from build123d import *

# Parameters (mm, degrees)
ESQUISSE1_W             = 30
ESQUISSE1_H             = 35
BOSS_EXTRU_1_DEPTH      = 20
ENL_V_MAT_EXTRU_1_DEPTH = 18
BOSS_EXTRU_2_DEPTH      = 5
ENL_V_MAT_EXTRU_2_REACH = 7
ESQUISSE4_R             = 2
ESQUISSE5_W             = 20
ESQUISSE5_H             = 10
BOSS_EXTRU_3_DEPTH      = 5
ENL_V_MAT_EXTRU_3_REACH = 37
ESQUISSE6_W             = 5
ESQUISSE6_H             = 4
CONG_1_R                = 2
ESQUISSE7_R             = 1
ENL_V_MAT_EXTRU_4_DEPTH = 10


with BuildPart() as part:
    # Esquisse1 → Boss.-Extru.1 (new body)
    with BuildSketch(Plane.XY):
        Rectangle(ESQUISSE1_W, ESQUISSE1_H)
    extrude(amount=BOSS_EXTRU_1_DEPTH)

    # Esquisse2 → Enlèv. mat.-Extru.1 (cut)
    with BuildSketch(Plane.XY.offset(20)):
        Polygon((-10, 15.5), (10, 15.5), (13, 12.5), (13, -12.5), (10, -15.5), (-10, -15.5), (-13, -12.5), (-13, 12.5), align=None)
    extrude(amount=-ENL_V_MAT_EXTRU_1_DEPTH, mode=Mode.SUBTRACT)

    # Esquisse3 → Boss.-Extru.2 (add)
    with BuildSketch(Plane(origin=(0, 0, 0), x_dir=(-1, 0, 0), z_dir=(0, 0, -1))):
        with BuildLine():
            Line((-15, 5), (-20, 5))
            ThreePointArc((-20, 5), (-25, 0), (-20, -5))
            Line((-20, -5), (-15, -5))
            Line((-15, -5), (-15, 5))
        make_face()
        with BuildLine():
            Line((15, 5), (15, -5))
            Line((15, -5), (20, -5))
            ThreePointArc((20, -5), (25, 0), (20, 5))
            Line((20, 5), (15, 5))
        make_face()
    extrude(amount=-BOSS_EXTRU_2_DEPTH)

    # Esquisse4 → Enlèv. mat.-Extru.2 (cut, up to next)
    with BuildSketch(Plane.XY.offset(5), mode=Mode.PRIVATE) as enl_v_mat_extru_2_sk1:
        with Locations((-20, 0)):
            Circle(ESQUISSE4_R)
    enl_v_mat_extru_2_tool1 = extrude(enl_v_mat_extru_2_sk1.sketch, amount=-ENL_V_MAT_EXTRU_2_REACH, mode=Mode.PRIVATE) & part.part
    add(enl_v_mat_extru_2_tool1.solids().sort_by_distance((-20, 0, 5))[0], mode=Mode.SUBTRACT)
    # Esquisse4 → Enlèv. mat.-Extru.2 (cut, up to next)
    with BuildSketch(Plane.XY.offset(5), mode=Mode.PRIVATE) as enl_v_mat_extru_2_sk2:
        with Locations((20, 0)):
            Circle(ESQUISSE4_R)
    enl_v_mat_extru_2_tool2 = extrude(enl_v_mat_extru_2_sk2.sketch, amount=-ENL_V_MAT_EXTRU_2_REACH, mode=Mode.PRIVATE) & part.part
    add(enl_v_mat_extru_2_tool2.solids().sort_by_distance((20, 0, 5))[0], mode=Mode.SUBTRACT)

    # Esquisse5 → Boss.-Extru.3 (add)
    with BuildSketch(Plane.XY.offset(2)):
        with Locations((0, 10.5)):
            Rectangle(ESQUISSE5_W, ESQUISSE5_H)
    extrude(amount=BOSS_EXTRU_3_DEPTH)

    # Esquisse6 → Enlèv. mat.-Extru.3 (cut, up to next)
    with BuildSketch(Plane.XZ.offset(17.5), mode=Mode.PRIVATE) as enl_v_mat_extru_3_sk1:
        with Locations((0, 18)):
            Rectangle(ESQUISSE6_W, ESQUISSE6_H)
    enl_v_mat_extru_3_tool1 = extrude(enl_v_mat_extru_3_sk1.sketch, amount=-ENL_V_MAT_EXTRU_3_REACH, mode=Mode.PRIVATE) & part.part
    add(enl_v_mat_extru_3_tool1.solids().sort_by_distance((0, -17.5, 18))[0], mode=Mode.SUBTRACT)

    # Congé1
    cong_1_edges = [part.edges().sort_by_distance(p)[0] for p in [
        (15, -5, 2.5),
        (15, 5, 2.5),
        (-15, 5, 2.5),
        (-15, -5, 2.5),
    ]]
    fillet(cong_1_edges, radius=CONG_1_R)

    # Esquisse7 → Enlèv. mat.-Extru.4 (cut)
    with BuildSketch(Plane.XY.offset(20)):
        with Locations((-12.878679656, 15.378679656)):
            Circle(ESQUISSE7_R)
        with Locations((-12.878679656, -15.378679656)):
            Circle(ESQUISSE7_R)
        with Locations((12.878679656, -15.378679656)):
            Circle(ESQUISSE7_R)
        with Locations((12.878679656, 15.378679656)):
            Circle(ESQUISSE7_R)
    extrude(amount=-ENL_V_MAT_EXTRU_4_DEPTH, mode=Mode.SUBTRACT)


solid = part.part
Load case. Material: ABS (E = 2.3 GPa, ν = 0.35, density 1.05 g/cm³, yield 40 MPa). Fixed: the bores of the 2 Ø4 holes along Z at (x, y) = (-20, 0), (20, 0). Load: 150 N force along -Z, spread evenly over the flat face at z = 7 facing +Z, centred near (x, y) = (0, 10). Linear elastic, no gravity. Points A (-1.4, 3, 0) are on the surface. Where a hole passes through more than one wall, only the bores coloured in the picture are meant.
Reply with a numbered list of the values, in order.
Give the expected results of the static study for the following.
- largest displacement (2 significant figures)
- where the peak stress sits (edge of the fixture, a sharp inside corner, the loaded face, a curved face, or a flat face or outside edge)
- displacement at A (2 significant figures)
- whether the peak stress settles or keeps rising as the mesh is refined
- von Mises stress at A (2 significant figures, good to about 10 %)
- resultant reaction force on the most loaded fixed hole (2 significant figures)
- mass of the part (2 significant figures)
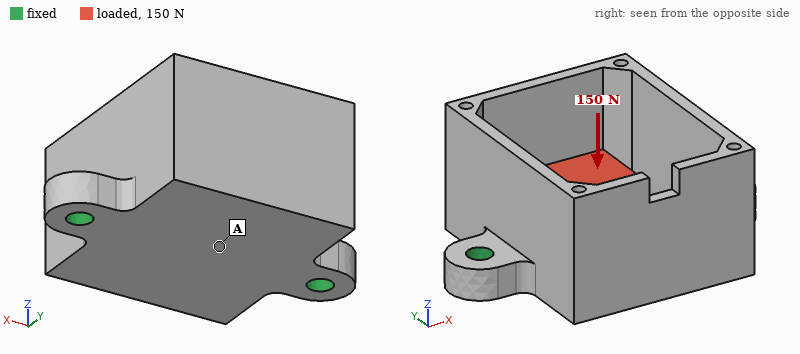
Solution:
1. 0.43 mm
2. edge of the fixture
3. 0.14 mm
4. keeps rising
5. 3.1 MPa
6. 76 N
7. 8.9 g
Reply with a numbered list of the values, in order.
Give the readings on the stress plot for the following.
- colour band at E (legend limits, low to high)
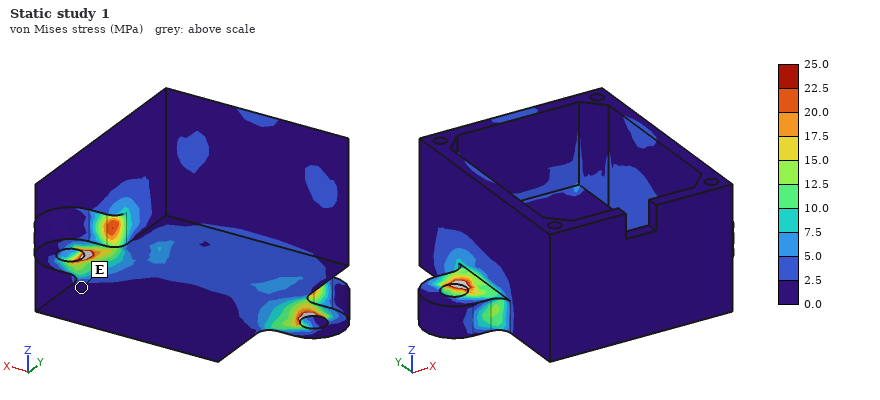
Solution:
1. 0.0 to 2.5 MPa
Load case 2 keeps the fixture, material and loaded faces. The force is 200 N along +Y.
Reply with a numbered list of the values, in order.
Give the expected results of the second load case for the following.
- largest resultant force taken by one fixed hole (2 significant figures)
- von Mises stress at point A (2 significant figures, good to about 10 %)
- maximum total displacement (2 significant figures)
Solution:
1. 100 N
2. 3.4 MPa
3. 0.31 mm
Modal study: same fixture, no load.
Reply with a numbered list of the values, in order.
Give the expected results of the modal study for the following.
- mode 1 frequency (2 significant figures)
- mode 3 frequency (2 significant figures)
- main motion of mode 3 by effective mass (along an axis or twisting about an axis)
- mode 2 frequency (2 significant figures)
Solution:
1. 1200 Hz
2. 3000 Hz
3. along Z
4. 2100 Hz
